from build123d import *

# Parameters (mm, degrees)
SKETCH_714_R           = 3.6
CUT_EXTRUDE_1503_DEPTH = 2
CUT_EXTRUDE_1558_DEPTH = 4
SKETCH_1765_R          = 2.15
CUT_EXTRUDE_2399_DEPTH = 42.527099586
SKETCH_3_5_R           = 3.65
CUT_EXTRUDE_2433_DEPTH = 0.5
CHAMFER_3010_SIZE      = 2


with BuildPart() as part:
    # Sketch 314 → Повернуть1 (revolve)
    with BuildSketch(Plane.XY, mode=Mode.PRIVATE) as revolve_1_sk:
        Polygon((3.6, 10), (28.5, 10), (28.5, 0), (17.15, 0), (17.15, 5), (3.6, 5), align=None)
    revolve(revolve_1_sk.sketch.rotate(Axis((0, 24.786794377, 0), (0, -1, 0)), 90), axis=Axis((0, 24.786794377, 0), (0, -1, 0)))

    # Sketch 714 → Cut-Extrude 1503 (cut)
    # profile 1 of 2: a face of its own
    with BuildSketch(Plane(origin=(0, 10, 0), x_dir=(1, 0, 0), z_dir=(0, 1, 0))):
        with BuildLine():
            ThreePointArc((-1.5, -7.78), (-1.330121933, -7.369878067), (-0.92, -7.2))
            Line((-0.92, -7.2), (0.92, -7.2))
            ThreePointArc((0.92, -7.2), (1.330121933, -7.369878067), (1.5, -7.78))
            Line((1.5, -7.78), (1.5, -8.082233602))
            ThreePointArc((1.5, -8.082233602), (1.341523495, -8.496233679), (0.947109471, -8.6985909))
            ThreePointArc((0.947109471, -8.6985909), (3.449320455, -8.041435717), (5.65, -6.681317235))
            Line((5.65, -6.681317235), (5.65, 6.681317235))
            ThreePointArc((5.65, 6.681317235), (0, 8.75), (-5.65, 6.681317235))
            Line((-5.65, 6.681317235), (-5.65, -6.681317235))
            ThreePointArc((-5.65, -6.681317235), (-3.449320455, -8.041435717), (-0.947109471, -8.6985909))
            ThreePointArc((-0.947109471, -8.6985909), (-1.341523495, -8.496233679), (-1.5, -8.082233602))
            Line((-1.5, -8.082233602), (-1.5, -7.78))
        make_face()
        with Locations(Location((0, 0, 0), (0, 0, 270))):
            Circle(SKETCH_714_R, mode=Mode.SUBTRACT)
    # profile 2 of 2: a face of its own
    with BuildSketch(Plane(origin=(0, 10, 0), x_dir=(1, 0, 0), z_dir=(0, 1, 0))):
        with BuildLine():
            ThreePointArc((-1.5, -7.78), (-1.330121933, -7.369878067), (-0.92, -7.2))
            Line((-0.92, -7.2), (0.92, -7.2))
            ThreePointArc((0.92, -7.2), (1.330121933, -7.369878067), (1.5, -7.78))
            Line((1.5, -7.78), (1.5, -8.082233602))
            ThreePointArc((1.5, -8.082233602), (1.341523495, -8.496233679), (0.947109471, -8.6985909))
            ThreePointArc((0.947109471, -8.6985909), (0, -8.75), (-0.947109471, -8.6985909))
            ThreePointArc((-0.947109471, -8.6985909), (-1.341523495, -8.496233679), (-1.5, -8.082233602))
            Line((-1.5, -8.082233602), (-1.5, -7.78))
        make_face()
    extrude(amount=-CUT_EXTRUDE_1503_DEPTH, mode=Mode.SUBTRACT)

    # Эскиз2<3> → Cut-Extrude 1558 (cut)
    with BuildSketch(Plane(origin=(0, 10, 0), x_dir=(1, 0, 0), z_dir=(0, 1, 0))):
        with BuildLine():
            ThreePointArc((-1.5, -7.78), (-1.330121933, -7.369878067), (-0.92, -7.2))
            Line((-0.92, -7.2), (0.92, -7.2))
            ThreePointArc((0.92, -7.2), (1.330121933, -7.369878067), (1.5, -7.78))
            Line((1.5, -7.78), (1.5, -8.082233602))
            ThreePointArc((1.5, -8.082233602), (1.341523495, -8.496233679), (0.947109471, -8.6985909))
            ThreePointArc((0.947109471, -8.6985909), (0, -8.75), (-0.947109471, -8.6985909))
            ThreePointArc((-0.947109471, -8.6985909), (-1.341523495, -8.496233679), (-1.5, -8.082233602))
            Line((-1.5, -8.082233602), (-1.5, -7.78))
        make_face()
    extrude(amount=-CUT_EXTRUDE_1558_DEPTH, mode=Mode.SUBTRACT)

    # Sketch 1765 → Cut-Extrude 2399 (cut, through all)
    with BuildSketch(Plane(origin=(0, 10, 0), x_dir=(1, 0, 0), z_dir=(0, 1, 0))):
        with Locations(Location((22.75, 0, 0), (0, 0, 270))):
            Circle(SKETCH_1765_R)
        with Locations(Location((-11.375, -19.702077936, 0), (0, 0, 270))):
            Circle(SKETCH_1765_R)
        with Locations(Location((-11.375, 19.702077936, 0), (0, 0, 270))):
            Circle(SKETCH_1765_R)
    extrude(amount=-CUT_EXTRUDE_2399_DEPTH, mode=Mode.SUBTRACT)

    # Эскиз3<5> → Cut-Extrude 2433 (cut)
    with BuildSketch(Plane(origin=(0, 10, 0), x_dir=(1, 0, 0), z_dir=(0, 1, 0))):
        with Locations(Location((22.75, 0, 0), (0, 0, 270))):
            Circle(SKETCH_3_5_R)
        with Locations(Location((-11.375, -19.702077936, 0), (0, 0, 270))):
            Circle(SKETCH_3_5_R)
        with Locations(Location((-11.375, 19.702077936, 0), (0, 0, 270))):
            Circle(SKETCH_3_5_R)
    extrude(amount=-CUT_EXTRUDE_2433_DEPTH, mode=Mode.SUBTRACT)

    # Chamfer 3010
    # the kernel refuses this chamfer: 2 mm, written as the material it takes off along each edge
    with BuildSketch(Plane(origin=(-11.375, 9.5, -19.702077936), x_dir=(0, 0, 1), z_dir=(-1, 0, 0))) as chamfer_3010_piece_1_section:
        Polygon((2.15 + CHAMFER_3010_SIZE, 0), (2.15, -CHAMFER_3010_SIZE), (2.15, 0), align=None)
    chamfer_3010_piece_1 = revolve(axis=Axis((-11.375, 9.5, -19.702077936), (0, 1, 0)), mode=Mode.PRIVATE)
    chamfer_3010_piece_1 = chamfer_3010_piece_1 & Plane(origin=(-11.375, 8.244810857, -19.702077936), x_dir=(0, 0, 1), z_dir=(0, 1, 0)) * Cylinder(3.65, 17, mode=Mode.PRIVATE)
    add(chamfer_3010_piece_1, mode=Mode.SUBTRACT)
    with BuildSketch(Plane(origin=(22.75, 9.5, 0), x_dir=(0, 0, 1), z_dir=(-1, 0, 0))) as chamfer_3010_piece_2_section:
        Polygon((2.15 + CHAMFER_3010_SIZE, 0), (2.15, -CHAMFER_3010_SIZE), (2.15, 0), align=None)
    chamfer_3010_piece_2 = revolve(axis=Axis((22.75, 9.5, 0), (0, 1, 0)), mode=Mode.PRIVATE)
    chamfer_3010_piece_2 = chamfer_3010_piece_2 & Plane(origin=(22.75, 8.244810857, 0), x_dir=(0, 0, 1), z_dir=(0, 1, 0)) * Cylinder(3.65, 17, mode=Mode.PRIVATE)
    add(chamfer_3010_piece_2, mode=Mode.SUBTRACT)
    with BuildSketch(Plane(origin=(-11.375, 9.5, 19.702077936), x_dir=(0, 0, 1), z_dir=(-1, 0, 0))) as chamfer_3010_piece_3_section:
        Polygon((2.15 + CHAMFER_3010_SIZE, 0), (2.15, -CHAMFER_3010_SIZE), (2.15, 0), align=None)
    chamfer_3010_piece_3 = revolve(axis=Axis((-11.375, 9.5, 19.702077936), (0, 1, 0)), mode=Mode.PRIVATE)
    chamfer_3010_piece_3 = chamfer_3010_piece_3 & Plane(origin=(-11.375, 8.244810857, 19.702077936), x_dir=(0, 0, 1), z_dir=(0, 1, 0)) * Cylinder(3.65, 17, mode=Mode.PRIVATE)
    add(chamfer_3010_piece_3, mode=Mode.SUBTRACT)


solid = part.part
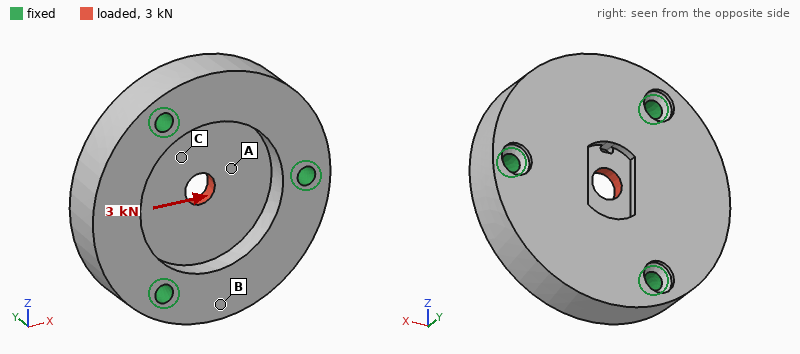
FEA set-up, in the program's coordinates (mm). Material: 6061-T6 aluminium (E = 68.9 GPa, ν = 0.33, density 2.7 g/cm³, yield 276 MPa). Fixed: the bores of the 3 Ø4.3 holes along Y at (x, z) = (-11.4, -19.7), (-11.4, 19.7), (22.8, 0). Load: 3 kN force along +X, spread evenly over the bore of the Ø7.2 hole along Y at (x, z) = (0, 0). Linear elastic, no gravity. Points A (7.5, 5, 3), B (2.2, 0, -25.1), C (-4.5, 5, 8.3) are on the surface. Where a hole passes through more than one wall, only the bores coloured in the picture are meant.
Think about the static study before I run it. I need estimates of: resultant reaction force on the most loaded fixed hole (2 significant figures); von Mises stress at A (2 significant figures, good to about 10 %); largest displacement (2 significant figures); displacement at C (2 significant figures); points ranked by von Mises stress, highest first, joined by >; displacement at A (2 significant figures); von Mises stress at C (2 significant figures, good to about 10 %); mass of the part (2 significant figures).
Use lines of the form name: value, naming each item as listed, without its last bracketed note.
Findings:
resultant reaction force on the most loaded fixed hole: 1.0 kN
von Mises stress at A: 34 MPa
largest displacement: 8.4 µm
displacement at C: 3.6 µm
points ranked by von Mises stress, highest first, joined by >: A > C > B
displacement at A: 4.8 µm
von Mises stress at C: 18 MPa
mass of the part: 54 g
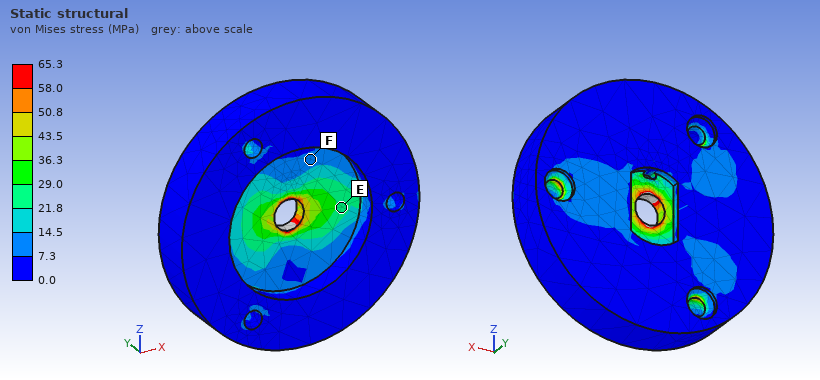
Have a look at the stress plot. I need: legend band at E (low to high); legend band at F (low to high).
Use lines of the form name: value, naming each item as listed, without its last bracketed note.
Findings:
legend band at E: 21.8 to 29.0 MPa
legend band at F: 7.3 to 14.5 MPa
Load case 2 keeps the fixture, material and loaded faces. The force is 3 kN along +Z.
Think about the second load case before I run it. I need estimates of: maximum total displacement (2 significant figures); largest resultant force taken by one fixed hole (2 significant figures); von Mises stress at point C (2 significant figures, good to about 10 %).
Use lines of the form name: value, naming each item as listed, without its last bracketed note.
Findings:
maximum total displacement: 8.3 µm
largest resultant force taken by one fixed hole: 1.0 kN
von Mises stress at point C: 27 MPa
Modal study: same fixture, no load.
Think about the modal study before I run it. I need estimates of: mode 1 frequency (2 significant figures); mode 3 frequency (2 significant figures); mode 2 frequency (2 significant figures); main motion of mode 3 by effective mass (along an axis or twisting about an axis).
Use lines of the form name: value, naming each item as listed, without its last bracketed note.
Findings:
mode 1 frequency: 14 kHz
mode 3 frequency: 17 kHz
mode 2 frequency: 14 kHz
main motion of mode 3 by effective mass: along Y
